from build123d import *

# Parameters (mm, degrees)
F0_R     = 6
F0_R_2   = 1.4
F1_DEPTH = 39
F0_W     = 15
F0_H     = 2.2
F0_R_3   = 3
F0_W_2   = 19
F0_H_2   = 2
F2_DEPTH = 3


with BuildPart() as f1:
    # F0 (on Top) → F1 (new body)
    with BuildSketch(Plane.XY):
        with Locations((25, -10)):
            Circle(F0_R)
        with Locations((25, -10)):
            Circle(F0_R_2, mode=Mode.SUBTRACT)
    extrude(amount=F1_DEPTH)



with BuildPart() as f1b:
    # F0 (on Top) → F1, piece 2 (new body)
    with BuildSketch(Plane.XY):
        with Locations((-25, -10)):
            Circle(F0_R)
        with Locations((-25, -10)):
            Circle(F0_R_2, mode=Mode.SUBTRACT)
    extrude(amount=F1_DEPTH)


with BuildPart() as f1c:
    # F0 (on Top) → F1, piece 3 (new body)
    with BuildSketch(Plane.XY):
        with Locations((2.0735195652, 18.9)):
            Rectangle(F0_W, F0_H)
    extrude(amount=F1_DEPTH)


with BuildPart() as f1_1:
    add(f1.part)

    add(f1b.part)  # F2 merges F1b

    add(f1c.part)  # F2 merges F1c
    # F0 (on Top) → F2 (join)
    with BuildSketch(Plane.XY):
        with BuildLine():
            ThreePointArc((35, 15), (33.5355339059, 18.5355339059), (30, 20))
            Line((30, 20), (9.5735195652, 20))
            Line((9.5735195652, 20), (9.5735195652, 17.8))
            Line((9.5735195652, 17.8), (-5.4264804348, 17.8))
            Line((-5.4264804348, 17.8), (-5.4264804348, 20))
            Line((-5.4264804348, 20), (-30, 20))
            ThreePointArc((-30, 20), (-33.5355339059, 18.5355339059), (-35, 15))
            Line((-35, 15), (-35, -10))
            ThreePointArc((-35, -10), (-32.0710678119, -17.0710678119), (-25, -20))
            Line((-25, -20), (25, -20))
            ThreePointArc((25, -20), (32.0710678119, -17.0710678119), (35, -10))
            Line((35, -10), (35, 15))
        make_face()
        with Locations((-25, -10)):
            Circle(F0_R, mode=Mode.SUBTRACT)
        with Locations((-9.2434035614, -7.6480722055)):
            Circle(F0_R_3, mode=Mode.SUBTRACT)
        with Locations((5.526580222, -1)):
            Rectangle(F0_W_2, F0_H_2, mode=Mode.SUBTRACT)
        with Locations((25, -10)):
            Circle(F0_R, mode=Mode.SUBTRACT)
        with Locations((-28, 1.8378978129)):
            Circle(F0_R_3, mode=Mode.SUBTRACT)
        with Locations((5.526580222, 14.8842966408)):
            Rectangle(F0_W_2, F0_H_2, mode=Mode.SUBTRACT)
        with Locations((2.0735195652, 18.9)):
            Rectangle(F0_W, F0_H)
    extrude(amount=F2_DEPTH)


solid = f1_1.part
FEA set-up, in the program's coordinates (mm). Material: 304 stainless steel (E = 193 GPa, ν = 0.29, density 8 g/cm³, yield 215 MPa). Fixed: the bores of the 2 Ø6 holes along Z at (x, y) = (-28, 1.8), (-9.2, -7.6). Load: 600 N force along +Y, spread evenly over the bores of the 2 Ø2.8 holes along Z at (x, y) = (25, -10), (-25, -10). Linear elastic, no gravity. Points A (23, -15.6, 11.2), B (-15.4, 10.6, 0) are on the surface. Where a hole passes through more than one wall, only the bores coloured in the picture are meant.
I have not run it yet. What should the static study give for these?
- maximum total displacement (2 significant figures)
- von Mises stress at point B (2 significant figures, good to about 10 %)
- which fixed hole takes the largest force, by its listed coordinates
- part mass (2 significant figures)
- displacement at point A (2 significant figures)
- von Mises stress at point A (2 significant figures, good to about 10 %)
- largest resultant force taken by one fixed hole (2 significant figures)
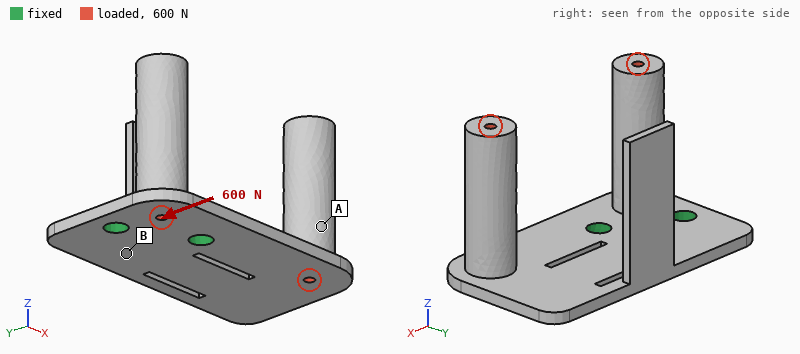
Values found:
0.30 mm
45 MPa
(-9.2, -7.6)
130 g
0.10 mm
17 MPa
700 N
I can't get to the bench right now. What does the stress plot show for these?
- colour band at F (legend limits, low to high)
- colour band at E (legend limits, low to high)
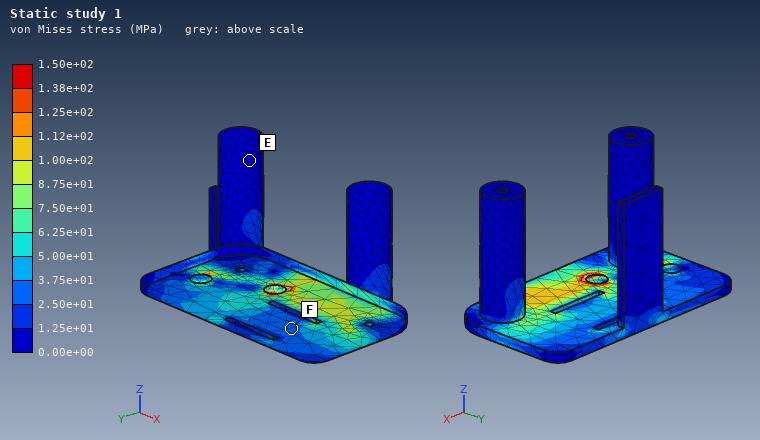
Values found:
2.50e+01 to 3.75e+01 MPa
0.00e+00 to 1.25e+01 MPa
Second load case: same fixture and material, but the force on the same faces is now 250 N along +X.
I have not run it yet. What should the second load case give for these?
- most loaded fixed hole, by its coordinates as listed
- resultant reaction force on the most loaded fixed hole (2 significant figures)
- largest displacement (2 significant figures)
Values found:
(-9.2, -7.6)
250 N
0.21 mm
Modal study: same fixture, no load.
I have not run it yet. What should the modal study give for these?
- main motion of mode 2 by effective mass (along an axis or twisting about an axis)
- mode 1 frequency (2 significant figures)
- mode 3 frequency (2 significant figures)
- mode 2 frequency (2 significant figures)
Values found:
along Y
590 Hz
1100 Hz
850 Hz
